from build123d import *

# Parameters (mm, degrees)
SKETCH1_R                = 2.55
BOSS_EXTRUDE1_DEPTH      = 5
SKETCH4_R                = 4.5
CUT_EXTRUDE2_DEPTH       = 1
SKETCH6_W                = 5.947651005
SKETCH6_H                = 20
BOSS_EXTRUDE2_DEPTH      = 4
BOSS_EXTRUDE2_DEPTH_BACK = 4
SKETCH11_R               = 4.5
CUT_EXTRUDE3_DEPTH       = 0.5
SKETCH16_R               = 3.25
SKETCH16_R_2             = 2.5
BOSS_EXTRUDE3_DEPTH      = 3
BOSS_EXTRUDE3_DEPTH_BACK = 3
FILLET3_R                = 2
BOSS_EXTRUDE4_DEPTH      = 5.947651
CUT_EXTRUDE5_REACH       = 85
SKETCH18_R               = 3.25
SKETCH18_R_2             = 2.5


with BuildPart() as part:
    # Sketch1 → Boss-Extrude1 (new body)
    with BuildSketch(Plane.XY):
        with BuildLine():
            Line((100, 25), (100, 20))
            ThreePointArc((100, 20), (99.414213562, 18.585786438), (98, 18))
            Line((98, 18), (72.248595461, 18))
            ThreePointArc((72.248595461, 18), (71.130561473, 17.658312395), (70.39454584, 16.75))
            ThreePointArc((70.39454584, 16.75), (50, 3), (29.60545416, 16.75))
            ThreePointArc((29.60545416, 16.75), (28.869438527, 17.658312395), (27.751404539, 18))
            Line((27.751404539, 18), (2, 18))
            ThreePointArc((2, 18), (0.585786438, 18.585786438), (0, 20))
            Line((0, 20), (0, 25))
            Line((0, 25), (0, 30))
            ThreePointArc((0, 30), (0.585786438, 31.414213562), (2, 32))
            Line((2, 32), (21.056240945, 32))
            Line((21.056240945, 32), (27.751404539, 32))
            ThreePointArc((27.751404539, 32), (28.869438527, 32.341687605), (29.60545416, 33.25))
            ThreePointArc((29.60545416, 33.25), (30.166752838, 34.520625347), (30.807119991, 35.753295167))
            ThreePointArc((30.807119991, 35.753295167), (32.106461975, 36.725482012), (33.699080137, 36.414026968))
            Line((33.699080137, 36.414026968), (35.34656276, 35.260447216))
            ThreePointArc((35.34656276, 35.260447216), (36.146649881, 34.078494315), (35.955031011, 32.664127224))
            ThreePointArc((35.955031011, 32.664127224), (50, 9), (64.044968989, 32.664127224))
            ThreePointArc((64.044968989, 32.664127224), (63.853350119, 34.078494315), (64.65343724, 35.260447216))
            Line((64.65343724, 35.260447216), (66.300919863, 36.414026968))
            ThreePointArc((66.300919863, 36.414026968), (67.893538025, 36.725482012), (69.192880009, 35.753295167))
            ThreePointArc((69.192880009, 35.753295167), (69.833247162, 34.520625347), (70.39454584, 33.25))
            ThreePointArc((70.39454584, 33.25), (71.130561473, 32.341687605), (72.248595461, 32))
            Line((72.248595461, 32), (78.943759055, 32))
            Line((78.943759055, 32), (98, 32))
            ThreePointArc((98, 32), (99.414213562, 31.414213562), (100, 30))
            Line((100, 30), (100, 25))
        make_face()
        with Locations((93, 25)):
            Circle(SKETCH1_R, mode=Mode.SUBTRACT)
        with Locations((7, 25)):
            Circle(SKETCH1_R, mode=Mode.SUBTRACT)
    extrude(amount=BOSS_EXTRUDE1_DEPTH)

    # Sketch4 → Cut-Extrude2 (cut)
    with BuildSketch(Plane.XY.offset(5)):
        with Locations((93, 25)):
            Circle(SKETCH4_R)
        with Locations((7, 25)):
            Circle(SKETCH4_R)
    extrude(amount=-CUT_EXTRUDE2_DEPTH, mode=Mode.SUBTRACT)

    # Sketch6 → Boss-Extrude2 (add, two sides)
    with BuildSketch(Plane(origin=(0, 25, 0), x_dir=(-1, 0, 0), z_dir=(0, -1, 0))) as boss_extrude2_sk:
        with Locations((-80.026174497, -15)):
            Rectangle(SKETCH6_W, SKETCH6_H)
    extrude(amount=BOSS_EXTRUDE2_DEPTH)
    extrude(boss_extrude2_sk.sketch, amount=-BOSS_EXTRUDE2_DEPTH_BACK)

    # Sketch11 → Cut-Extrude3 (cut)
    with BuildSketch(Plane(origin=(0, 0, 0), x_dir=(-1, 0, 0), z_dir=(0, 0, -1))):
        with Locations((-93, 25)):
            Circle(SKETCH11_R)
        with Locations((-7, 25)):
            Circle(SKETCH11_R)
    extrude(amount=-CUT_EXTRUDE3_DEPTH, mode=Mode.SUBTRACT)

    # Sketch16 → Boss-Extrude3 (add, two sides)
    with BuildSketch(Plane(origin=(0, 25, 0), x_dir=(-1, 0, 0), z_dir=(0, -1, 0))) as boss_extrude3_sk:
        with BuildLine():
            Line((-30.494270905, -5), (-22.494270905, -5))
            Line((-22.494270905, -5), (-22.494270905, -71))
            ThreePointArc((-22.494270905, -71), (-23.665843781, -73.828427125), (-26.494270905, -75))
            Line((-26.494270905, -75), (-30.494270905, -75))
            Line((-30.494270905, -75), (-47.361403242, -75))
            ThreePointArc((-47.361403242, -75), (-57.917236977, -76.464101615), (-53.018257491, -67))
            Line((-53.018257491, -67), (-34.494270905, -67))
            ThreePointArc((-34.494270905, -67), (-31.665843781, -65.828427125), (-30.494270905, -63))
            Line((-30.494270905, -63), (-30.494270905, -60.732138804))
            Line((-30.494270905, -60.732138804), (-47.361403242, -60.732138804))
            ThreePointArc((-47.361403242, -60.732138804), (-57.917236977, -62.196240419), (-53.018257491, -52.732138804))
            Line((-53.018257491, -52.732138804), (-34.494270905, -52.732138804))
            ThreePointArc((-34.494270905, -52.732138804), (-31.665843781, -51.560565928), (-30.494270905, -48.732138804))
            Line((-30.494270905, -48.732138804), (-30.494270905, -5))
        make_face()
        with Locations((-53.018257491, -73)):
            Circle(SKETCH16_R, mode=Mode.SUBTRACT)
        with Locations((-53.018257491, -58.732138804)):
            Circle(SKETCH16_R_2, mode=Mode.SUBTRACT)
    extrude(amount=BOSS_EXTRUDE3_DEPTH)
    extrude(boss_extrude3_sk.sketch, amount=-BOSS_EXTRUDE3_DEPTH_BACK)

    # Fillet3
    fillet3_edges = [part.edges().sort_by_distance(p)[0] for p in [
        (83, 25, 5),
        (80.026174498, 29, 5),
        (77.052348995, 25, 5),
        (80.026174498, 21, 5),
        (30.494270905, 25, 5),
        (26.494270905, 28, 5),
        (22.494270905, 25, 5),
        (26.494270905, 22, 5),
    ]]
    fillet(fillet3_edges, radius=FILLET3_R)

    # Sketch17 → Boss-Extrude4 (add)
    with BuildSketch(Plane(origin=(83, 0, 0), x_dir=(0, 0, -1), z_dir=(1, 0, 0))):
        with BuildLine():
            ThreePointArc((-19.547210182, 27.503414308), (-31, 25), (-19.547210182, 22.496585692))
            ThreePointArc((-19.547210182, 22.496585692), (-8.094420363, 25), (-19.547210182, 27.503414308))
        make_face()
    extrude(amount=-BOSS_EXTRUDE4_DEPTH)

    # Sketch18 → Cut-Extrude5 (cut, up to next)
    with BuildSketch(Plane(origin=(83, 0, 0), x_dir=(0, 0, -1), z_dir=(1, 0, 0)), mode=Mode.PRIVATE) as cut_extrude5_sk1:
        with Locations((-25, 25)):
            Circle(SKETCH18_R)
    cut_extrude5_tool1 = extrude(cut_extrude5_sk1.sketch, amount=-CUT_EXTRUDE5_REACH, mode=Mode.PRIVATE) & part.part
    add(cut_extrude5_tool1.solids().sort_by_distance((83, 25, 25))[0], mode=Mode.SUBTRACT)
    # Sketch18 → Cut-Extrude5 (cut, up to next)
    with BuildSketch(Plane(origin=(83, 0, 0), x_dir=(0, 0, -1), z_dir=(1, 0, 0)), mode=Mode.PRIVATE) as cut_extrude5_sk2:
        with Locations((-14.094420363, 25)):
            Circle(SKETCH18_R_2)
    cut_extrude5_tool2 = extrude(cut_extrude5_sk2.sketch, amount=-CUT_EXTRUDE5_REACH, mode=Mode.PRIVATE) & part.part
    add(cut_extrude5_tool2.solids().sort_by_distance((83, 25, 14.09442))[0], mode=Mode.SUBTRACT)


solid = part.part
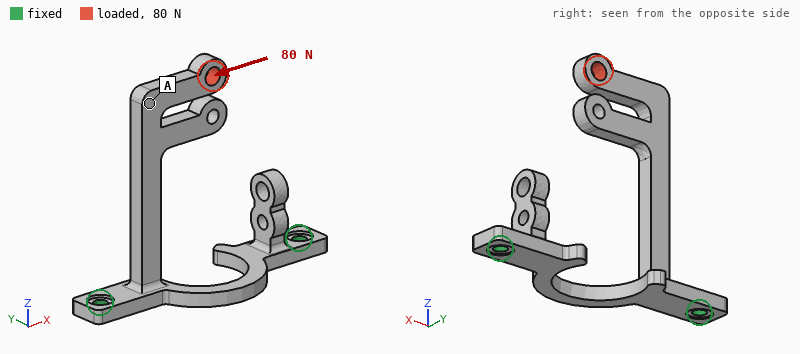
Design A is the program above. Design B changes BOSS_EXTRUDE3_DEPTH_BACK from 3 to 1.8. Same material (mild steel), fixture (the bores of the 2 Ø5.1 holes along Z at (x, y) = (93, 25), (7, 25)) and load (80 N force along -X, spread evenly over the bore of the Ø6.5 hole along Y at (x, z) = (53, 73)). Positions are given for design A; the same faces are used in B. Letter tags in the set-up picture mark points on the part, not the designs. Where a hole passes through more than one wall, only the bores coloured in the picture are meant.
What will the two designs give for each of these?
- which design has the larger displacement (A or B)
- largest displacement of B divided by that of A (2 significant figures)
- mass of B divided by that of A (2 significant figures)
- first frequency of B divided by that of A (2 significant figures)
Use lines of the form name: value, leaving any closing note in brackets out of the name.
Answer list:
which design has the larger displacement: B
largest displacement of B divided by that of A: 1.1
mass of B divided by that of A: 0.91
first frequency of B divided by that of A: 0.90
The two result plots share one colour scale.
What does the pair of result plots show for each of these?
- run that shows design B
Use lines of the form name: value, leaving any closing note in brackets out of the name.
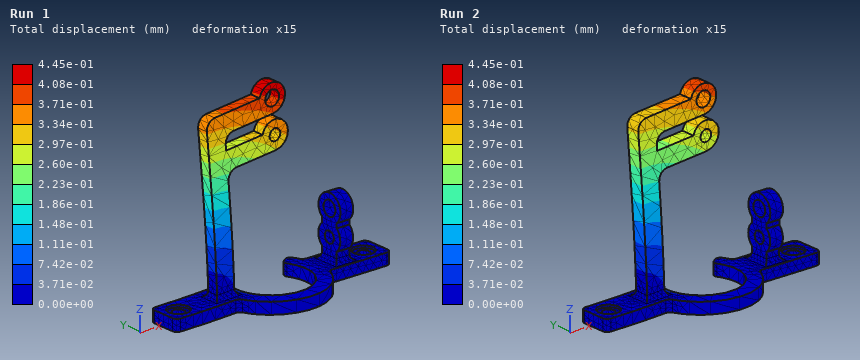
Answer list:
run that shows design B: Run 1
